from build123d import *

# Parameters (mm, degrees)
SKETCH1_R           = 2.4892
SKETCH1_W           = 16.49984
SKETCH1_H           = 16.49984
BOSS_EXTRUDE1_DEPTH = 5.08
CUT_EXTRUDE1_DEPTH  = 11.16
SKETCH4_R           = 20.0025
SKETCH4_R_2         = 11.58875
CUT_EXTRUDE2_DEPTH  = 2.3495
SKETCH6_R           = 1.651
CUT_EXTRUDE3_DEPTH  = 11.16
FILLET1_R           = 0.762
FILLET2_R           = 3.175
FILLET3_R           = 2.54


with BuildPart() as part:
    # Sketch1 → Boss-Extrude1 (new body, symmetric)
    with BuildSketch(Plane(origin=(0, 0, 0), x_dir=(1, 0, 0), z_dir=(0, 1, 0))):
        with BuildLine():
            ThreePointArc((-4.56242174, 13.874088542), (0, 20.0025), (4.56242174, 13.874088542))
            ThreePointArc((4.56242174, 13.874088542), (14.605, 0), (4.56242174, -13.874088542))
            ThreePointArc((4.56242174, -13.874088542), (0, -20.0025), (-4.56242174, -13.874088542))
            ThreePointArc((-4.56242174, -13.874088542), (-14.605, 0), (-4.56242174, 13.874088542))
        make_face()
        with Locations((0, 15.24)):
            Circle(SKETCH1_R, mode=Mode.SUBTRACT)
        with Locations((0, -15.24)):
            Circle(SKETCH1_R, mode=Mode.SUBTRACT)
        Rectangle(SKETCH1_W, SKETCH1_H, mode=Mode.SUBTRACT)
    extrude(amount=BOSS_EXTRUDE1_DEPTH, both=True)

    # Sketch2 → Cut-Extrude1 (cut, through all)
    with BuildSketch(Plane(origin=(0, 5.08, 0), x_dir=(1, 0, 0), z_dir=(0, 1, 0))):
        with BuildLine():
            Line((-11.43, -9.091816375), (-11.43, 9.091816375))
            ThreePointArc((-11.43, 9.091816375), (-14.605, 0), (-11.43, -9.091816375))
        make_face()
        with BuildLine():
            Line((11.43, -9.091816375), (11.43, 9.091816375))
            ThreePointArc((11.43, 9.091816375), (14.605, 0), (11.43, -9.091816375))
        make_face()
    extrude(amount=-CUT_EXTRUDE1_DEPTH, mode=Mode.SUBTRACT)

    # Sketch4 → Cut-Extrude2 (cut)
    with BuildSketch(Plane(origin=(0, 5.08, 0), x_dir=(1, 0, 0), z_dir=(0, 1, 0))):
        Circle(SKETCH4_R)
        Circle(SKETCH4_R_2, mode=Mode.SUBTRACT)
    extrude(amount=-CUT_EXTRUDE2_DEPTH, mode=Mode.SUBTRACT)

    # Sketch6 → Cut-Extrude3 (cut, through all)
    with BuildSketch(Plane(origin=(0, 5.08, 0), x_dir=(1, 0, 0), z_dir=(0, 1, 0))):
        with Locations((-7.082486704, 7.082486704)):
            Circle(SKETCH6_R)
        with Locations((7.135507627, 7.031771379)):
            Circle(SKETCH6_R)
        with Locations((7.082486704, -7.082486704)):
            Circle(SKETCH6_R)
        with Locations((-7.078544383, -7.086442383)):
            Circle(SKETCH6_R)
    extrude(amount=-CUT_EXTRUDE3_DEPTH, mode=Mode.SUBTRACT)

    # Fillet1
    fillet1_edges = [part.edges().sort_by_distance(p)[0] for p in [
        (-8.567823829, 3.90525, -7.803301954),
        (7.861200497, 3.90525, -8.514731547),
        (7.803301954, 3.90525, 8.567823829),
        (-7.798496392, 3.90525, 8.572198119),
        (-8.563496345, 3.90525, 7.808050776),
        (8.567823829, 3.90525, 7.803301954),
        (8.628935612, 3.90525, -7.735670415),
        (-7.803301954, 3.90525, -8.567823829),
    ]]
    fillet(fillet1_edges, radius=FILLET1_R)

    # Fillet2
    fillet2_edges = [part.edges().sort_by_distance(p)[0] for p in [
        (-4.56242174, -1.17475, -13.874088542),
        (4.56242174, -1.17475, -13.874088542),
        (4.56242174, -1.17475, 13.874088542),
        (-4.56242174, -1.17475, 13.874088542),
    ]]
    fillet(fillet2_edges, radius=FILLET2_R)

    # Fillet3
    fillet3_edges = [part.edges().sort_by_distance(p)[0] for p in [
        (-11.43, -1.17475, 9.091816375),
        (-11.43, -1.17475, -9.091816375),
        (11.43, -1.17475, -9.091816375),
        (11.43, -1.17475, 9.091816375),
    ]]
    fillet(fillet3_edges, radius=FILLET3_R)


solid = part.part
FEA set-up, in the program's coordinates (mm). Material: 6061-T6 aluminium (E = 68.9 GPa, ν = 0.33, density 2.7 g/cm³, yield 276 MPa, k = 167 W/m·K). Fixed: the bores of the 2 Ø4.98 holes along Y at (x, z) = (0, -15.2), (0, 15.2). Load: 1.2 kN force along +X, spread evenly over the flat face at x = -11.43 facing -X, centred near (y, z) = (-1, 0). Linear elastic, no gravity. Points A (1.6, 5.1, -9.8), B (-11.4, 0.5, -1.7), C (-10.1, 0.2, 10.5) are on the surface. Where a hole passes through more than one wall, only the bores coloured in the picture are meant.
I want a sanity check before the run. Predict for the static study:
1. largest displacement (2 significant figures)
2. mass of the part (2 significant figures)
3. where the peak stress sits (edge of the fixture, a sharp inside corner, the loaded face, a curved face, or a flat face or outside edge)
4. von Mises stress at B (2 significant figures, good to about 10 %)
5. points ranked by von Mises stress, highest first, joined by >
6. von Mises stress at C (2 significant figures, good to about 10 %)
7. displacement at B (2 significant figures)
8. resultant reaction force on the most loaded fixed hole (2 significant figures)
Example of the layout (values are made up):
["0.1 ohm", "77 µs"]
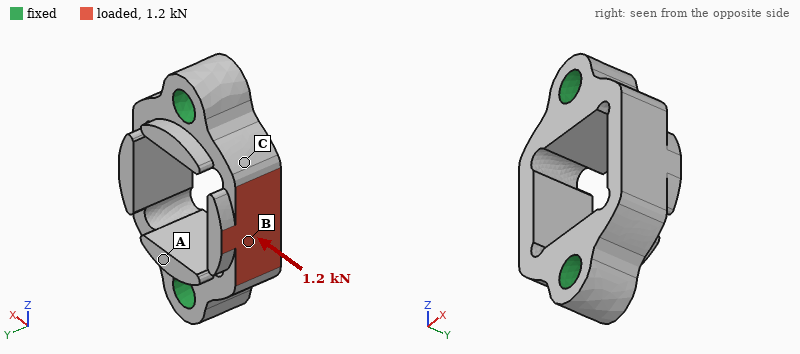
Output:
["40 µm", "8.6 g", "a curved face", "110 MPa", "B > C > A", "54 MPa", "33 µm", "760 N"]
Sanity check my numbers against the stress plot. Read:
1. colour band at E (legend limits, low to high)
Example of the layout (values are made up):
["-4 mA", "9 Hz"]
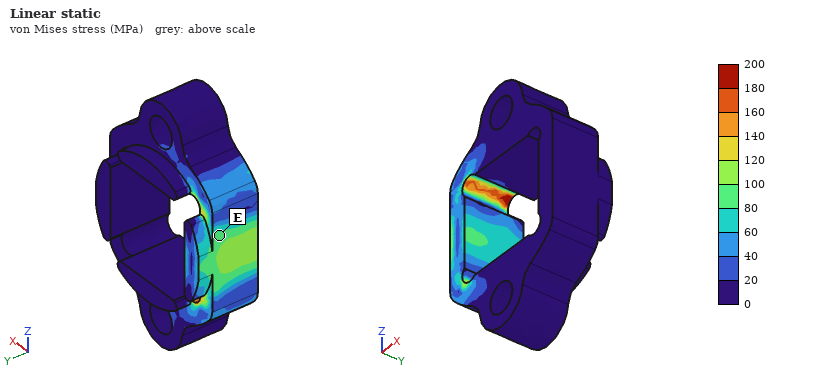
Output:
["80 to 100 MPa"]
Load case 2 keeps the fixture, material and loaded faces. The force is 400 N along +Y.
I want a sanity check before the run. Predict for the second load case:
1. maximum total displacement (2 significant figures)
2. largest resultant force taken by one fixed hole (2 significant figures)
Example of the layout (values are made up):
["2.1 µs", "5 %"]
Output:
["17 µm", "200 N"]
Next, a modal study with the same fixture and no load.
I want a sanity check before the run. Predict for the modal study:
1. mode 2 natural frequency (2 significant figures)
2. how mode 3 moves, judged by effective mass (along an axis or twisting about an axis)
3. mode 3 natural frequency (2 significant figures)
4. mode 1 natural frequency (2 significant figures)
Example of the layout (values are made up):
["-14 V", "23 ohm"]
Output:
["26 kHz", "along X", "28 kHz", "25 kHz"]
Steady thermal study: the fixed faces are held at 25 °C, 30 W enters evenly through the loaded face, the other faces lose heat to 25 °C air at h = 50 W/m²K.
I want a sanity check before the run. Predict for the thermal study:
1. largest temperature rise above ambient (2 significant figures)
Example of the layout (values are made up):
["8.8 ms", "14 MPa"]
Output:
["42 K"]
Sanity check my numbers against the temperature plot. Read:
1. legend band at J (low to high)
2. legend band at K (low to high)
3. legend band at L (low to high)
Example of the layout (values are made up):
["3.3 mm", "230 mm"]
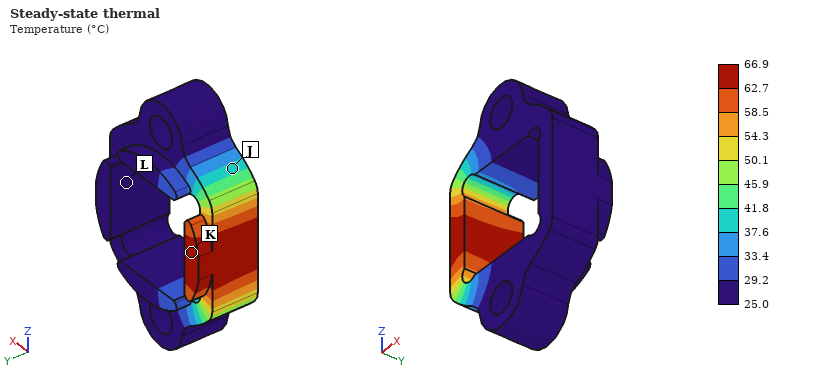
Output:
["37.6 to 41.8 °C", "62.7 to 66.9 °C", "25.0 to 29.2 °C"]
